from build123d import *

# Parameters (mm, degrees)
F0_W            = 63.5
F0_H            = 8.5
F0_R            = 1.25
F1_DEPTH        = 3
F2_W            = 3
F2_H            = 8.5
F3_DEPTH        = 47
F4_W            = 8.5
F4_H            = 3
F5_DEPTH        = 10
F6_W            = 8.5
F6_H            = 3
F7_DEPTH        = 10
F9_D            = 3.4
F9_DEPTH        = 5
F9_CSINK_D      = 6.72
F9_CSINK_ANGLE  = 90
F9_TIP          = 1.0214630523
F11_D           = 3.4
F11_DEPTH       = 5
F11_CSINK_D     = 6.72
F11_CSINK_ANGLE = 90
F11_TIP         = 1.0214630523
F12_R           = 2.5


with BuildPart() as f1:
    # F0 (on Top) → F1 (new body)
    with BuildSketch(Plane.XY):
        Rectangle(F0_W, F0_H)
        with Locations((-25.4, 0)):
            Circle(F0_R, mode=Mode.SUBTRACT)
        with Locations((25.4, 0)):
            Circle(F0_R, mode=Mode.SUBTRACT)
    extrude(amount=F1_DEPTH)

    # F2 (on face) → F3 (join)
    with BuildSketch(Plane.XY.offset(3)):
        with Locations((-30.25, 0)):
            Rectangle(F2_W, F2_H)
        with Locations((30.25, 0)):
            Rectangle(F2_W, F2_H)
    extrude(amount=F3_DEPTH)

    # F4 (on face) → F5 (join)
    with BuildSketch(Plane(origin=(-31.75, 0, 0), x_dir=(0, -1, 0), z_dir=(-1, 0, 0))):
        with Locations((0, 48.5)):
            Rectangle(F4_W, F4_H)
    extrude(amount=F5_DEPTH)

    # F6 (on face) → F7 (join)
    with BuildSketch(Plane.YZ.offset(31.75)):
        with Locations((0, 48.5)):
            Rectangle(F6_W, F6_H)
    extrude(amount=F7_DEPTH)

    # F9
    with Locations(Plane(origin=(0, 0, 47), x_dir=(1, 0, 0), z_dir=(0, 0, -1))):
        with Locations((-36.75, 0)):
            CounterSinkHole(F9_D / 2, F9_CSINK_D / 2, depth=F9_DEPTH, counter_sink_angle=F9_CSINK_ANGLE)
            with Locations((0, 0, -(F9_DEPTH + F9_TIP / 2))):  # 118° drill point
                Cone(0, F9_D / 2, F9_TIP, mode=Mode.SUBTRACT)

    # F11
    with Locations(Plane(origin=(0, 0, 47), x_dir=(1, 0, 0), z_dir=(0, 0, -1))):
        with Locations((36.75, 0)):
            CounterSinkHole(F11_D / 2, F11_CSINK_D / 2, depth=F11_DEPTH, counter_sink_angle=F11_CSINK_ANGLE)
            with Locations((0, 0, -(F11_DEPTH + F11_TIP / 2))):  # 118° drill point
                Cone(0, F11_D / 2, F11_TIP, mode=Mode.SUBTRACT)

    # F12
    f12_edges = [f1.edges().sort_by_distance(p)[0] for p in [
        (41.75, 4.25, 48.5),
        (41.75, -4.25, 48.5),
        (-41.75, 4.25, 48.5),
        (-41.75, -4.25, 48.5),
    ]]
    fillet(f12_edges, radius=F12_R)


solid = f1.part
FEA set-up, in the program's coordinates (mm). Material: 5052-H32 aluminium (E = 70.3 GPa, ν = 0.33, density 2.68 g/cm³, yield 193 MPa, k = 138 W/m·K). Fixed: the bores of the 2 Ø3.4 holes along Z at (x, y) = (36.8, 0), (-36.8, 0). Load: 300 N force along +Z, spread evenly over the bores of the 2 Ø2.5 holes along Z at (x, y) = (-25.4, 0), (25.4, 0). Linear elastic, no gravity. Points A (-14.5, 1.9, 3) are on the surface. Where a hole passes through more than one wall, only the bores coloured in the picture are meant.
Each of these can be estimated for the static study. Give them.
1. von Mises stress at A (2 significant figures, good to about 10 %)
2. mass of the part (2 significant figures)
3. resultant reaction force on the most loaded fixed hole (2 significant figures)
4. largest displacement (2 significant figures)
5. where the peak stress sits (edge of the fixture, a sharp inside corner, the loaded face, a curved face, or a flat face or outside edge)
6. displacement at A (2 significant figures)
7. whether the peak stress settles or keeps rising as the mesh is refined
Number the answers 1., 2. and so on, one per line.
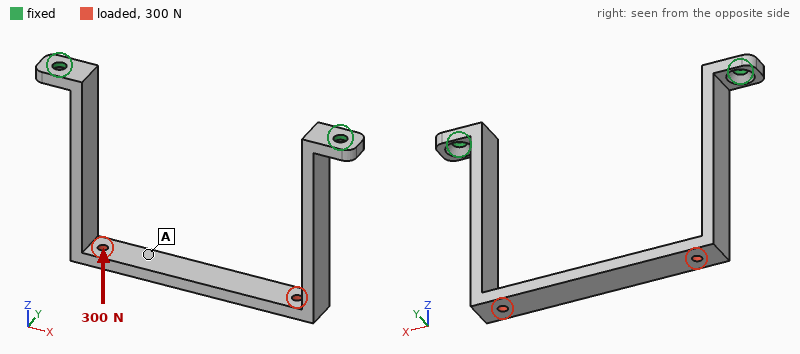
1. 15 MPa
2. 12 g
3. 150 N
4. 81 µm
5. edge of the fixture
6. 65 µm
7. keeps rising
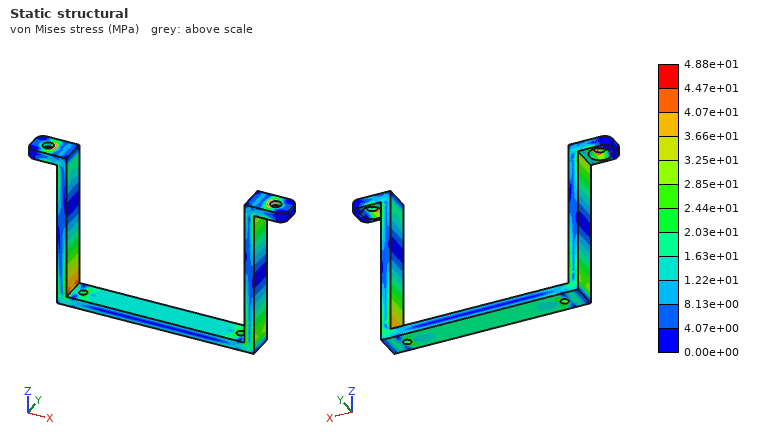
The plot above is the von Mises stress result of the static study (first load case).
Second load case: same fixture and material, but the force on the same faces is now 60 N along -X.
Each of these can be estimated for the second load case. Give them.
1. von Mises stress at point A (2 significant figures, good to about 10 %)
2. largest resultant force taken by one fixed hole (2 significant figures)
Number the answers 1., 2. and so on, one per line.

1. 26 MPa
2. 38 N
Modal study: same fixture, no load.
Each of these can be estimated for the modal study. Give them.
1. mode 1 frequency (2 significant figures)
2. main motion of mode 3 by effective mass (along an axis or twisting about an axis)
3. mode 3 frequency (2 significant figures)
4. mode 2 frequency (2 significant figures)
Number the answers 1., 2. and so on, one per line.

1. 780 Hz
2. twisting about Z
3. 1400 Hz
4. 800 Hz
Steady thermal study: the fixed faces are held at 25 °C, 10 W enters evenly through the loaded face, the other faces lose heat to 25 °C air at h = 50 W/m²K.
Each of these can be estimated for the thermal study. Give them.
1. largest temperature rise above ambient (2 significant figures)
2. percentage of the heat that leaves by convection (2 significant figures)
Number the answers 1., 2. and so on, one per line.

1. 46 K
2. 52 %
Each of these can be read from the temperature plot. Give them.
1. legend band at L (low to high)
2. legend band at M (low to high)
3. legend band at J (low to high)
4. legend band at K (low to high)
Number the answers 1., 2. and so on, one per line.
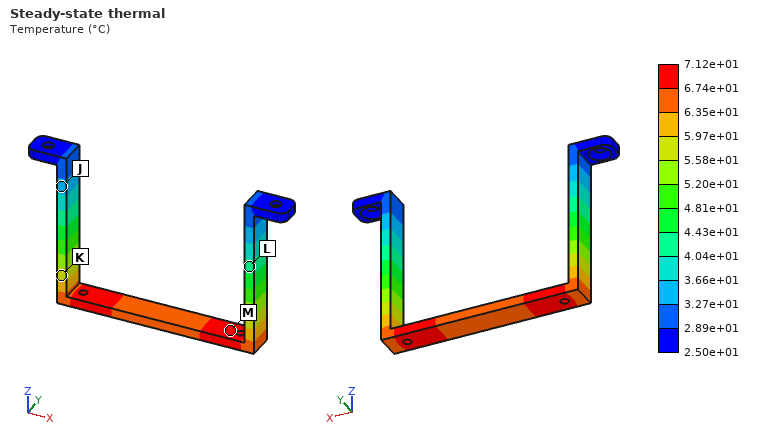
1. 4.04e+01 to 4.43e+01 °C
2. 6.74e+01 to 7.12e+01 °C
3. 3.27e+01 to 3.66e+01 °C
4. 5.58e+01 to 5.97e+01 °C
